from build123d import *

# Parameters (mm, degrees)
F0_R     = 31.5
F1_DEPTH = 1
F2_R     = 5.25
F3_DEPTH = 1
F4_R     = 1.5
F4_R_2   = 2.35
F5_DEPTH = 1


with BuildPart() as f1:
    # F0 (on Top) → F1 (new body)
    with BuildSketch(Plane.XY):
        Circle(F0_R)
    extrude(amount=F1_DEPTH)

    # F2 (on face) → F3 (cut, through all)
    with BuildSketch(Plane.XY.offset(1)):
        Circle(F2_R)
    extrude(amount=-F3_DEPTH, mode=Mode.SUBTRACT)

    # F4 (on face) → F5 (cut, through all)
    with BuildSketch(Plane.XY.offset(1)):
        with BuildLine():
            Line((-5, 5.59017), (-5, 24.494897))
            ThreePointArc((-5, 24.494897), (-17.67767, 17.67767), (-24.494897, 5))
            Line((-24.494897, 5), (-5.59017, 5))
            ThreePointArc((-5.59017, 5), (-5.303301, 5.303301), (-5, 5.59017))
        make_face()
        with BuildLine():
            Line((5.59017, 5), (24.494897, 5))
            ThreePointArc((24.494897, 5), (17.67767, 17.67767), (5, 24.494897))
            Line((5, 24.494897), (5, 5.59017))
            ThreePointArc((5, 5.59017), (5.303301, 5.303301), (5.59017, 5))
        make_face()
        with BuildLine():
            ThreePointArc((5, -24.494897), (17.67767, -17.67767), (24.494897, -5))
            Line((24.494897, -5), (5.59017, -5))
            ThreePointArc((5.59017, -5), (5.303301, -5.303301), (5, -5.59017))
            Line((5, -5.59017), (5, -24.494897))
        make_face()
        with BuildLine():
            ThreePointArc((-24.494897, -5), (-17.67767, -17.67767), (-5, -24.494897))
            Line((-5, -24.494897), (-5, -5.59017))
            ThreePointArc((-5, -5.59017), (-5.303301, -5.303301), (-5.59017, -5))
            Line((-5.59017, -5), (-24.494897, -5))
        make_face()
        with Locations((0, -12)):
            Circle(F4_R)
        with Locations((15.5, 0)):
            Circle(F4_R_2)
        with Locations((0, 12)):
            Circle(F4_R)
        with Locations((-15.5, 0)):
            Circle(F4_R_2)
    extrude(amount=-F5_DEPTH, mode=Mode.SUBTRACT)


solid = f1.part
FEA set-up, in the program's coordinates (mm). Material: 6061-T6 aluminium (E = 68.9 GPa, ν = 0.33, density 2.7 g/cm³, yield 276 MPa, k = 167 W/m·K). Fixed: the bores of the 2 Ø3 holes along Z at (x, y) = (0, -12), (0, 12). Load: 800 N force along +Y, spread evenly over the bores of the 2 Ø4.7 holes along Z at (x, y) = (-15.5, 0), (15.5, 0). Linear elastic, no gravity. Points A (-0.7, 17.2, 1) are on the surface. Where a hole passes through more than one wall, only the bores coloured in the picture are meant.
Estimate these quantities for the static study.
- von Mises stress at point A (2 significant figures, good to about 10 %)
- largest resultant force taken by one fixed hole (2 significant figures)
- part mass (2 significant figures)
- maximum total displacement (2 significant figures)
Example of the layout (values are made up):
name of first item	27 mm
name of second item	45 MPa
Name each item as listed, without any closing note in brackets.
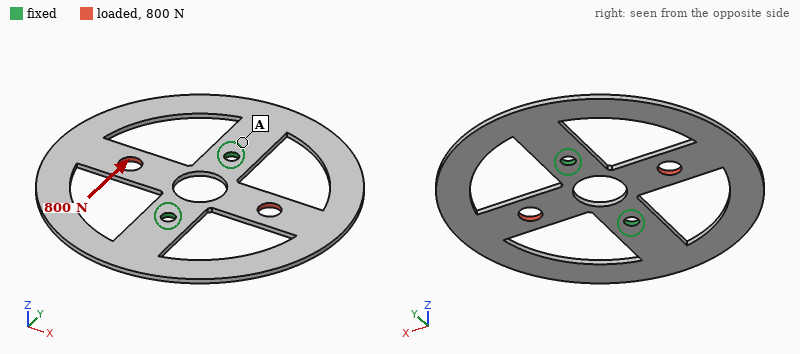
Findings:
von Mises stress at point A	18 MPa
largest resultant force taken by one fixed hole	400 N
part mass	5.2 g
maximum total displacement	41 µm
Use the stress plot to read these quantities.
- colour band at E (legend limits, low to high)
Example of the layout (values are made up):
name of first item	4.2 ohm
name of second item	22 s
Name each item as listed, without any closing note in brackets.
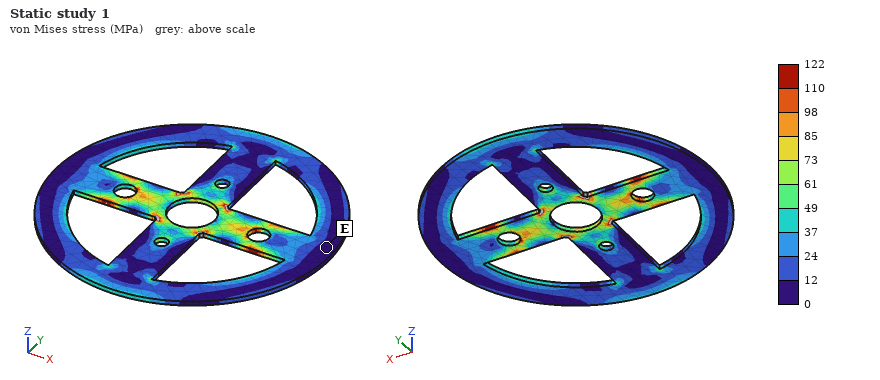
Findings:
colour band at E	0 to 12 MPa
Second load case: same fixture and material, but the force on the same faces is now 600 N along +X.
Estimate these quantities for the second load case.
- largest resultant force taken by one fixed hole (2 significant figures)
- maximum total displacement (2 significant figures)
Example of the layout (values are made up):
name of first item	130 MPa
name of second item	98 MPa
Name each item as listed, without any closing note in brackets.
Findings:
largest resultant force taken by one fixed hole	300 N
maximum total displacement	19 µm
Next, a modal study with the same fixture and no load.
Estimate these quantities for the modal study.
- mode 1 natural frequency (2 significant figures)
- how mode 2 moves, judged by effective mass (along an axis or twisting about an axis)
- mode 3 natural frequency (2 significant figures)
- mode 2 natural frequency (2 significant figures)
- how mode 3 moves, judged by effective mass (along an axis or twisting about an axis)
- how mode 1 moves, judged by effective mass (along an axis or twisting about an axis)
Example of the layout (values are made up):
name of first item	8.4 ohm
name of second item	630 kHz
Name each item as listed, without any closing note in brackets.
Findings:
mode 1 natural frequency	580 Hz
how mode 2 moves, judged by effective mass	along Z
mode 3 natural frequency	1300 Hz
mode 2 natural frequency	710 Hz
how mode 3 moves, judged by effective mass	twisting about X
how mode 1 moves, judged by effective mass	twisting about Y
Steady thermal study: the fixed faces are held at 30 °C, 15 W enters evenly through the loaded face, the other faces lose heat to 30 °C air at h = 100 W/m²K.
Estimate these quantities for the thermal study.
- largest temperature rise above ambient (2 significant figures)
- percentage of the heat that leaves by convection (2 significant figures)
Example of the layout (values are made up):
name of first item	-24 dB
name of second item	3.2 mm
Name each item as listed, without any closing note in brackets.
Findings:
largest temperature rise above ambient	47 K
percentage of the heat that leaves by convection	50 %
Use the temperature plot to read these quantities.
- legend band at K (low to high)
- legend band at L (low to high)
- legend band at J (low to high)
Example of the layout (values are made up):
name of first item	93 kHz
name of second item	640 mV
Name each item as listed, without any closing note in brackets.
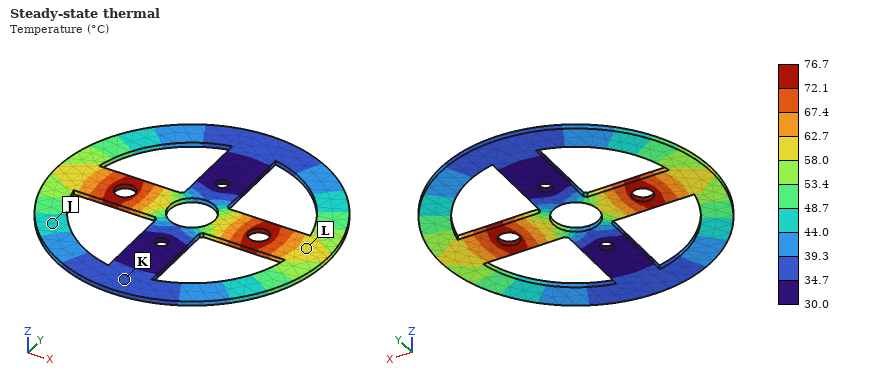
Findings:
legend band at K	34.7 to 39.3 °C
legend band at L	58.0 to 62.7 °C
legend band at J	44.0 to 48.7 °C
